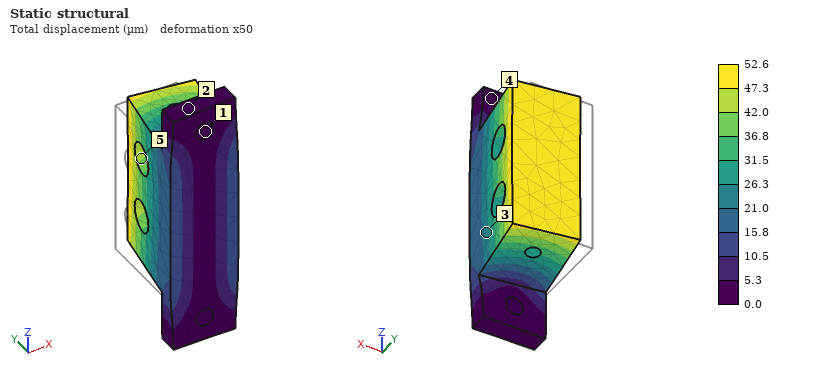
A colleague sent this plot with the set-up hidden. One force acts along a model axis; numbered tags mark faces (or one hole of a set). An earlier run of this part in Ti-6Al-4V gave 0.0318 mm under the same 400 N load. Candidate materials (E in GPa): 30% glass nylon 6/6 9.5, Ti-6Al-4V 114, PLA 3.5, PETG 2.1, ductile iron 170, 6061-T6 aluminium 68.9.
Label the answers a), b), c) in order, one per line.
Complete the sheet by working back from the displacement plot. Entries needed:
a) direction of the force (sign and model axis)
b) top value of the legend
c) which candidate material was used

a) +X
b) 52.6 µm
c) 6061-T6 aluminium
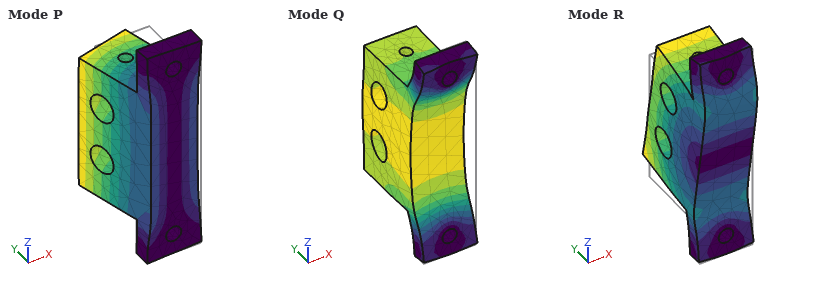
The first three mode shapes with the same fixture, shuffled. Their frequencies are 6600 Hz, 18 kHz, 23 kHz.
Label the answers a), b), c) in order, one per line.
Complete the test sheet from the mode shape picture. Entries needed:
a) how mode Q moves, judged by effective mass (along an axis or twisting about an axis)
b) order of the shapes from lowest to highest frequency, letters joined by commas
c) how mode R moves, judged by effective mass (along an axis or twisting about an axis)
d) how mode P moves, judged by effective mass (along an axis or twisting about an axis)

a) along Y
b) P, Q, R
c) along Z
d) along X
